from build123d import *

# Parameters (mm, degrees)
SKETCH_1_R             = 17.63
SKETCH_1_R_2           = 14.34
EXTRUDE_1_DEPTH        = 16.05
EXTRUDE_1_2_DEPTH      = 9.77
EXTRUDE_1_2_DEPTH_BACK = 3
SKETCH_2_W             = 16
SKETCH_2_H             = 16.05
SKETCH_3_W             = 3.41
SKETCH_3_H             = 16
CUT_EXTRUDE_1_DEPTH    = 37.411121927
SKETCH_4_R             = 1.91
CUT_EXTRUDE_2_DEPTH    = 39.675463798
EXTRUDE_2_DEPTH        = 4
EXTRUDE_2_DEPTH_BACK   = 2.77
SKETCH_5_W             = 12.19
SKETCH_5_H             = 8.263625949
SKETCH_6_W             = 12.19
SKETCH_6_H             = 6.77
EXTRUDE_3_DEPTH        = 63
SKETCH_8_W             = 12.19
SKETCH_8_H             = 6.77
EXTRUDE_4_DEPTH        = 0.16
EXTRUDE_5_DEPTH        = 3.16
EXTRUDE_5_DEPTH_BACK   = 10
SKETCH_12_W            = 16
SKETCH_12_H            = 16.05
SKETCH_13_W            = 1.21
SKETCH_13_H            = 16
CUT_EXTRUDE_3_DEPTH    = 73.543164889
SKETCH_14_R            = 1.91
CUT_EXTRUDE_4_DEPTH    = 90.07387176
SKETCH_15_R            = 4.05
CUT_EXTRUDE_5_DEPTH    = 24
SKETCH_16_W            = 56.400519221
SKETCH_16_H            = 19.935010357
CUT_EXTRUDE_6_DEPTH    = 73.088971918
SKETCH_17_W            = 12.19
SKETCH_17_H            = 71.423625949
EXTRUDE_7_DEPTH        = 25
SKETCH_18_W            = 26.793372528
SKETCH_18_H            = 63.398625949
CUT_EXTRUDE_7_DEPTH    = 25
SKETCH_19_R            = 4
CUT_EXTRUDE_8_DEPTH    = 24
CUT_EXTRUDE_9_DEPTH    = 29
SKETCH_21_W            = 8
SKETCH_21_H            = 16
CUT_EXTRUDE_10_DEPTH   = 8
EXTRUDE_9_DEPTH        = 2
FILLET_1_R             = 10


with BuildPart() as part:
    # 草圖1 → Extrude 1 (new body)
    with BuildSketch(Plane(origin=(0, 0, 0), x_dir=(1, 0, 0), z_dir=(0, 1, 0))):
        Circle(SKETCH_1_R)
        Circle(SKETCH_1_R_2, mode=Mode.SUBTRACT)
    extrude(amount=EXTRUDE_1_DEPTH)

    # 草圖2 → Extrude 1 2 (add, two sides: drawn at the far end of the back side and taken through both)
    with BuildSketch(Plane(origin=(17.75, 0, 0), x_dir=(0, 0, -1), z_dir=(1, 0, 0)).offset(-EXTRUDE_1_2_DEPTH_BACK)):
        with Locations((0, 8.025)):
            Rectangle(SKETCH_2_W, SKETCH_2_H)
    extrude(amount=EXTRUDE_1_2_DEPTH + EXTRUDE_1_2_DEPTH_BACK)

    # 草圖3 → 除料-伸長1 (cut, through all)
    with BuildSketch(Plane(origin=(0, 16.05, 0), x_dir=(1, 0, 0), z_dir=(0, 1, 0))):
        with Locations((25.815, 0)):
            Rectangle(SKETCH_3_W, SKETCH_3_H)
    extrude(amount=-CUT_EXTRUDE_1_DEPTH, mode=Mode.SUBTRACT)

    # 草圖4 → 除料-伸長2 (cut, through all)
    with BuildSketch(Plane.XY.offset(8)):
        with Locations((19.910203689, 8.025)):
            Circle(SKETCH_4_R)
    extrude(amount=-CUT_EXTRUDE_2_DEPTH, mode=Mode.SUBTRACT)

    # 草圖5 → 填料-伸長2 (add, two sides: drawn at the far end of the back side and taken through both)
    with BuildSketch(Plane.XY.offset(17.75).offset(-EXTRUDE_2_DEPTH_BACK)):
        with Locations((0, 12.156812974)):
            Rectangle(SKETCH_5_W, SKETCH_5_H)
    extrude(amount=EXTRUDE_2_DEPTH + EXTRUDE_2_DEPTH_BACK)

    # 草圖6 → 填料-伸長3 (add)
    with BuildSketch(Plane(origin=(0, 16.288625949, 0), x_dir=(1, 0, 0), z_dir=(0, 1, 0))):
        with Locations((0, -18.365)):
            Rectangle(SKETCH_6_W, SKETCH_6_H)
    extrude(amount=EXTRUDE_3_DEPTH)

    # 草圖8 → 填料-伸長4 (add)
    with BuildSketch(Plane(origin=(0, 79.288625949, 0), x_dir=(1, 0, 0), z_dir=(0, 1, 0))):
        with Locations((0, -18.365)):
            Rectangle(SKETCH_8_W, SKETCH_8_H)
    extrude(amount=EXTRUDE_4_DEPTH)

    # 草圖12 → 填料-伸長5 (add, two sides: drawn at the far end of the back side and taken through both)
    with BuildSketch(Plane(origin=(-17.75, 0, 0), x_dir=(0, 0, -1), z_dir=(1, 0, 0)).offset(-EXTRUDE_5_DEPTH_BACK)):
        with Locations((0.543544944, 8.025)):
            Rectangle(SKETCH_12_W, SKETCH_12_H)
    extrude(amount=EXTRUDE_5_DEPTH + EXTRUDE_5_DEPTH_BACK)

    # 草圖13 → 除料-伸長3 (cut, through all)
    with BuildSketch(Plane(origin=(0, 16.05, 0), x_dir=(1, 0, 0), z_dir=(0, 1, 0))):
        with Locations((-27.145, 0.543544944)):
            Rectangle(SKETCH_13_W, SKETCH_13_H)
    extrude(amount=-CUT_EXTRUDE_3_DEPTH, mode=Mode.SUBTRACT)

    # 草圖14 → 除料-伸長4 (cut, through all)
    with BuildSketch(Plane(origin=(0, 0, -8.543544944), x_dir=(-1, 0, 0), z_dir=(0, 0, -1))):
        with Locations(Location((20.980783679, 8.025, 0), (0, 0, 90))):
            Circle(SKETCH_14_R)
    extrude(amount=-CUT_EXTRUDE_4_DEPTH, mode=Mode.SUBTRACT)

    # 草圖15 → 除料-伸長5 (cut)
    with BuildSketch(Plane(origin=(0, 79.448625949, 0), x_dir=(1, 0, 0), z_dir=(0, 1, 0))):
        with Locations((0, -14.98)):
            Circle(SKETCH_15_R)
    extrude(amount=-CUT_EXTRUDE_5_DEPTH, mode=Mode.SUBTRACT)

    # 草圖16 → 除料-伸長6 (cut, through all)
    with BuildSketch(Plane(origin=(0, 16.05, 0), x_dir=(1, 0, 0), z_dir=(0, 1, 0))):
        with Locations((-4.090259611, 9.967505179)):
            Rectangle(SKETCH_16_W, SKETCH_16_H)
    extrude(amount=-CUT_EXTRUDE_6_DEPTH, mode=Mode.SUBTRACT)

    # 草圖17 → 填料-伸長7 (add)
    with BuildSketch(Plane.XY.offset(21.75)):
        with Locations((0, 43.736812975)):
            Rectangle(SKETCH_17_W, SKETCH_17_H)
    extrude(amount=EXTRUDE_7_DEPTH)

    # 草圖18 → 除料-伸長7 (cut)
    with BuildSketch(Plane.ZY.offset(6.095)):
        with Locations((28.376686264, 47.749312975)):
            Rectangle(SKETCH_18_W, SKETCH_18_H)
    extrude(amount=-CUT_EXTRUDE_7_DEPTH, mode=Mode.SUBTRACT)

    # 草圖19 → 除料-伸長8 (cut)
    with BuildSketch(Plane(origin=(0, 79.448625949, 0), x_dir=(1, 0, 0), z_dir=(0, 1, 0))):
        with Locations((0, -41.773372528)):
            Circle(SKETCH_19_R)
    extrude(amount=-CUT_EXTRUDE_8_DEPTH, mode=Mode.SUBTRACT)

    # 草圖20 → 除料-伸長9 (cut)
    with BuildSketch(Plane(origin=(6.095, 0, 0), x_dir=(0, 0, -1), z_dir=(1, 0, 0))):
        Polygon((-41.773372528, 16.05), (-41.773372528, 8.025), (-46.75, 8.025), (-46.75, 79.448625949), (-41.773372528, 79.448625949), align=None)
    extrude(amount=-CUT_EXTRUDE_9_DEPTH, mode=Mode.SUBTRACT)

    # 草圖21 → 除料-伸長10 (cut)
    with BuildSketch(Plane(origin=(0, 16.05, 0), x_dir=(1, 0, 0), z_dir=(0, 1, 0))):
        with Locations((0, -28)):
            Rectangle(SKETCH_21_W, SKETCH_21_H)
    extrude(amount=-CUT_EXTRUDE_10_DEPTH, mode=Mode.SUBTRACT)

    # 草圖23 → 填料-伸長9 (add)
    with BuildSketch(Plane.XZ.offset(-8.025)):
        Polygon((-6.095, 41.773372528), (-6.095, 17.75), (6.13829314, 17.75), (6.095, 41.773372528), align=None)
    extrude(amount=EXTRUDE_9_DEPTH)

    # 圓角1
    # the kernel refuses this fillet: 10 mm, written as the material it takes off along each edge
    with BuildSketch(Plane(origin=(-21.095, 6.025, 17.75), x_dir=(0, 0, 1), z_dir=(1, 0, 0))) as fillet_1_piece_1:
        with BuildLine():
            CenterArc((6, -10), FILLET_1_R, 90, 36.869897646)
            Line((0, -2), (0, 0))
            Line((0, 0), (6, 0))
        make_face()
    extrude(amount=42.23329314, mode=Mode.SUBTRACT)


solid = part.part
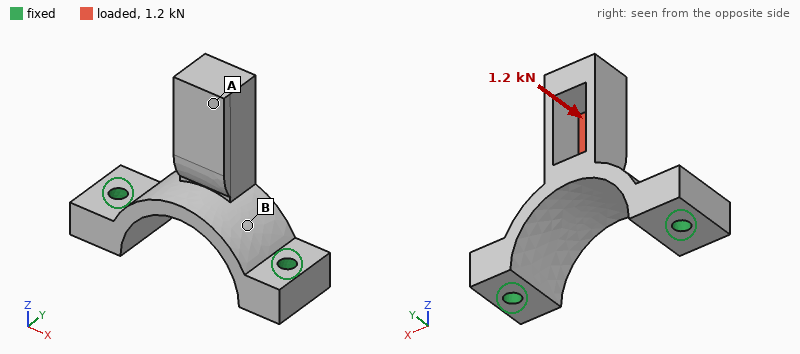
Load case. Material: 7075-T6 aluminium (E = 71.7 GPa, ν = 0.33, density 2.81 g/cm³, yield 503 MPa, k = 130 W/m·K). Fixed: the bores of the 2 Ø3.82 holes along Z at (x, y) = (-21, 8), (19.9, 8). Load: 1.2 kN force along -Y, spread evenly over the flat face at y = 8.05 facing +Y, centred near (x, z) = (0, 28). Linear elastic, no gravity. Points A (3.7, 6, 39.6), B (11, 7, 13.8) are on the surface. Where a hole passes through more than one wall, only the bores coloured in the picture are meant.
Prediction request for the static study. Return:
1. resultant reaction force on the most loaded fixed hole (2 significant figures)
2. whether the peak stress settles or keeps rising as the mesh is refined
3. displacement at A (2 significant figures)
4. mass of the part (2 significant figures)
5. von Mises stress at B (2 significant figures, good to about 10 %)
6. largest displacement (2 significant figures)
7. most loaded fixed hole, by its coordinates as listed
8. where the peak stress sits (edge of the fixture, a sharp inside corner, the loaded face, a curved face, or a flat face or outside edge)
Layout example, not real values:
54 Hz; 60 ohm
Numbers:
650 N; keeps rising; 0.38 mm; 18 g; 94 MPa; 0.41 mm; (19.9, 8); a sharp inside corner
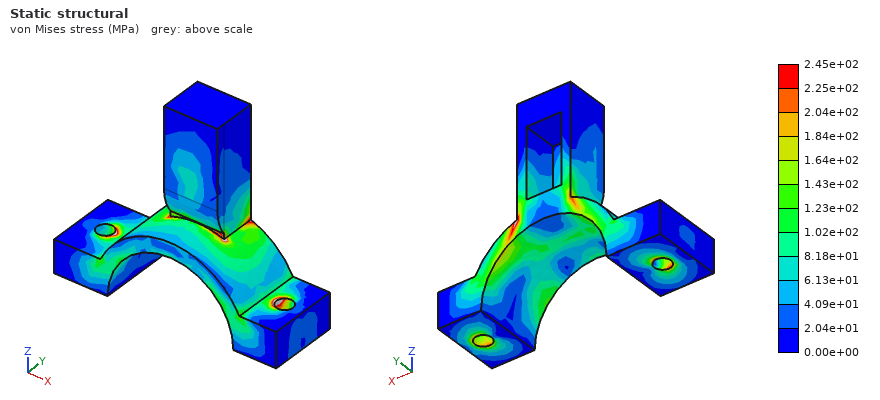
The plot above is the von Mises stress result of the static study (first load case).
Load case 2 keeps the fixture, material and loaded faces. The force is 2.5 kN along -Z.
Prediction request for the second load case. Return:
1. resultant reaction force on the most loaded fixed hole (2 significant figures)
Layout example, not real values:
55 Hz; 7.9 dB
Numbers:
1.8 kN
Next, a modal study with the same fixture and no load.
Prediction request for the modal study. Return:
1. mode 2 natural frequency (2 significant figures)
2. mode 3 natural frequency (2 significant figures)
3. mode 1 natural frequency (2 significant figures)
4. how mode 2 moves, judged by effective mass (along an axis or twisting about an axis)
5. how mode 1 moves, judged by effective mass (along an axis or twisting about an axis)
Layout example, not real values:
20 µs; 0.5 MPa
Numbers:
5700 Hz; 13 kHz; 3900 Hz; along X; along Y
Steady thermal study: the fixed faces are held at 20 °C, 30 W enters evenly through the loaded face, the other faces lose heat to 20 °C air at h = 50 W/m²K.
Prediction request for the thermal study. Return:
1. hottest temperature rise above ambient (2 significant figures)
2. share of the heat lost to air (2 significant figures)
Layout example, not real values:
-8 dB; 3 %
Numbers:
79 K; 20 %
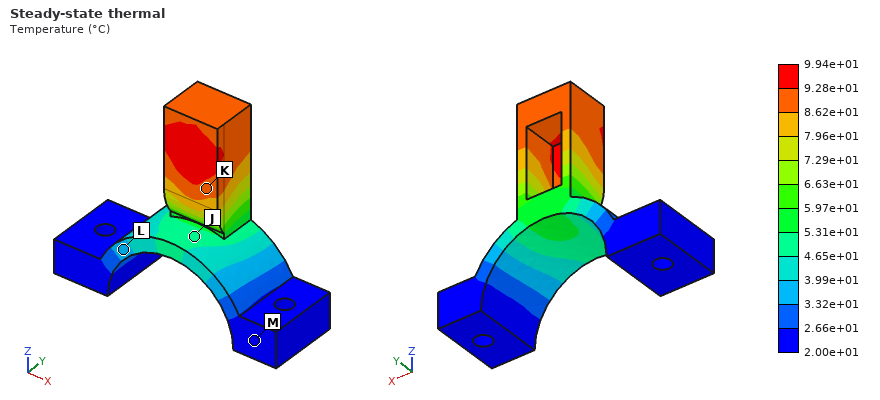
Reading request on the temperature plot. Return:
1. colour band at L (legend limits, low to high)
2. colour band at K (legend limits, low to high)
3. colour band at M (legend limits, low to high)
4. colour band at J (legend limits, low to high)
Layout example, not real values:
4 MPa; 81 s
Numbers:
3.32e+01 to 3.99e+01 °C; 8.62e+01 to 9.28e+01 °C; 2.00e+01 to 2.66e+01 °C; 4.65e+01 to 5.31e+01 °C
